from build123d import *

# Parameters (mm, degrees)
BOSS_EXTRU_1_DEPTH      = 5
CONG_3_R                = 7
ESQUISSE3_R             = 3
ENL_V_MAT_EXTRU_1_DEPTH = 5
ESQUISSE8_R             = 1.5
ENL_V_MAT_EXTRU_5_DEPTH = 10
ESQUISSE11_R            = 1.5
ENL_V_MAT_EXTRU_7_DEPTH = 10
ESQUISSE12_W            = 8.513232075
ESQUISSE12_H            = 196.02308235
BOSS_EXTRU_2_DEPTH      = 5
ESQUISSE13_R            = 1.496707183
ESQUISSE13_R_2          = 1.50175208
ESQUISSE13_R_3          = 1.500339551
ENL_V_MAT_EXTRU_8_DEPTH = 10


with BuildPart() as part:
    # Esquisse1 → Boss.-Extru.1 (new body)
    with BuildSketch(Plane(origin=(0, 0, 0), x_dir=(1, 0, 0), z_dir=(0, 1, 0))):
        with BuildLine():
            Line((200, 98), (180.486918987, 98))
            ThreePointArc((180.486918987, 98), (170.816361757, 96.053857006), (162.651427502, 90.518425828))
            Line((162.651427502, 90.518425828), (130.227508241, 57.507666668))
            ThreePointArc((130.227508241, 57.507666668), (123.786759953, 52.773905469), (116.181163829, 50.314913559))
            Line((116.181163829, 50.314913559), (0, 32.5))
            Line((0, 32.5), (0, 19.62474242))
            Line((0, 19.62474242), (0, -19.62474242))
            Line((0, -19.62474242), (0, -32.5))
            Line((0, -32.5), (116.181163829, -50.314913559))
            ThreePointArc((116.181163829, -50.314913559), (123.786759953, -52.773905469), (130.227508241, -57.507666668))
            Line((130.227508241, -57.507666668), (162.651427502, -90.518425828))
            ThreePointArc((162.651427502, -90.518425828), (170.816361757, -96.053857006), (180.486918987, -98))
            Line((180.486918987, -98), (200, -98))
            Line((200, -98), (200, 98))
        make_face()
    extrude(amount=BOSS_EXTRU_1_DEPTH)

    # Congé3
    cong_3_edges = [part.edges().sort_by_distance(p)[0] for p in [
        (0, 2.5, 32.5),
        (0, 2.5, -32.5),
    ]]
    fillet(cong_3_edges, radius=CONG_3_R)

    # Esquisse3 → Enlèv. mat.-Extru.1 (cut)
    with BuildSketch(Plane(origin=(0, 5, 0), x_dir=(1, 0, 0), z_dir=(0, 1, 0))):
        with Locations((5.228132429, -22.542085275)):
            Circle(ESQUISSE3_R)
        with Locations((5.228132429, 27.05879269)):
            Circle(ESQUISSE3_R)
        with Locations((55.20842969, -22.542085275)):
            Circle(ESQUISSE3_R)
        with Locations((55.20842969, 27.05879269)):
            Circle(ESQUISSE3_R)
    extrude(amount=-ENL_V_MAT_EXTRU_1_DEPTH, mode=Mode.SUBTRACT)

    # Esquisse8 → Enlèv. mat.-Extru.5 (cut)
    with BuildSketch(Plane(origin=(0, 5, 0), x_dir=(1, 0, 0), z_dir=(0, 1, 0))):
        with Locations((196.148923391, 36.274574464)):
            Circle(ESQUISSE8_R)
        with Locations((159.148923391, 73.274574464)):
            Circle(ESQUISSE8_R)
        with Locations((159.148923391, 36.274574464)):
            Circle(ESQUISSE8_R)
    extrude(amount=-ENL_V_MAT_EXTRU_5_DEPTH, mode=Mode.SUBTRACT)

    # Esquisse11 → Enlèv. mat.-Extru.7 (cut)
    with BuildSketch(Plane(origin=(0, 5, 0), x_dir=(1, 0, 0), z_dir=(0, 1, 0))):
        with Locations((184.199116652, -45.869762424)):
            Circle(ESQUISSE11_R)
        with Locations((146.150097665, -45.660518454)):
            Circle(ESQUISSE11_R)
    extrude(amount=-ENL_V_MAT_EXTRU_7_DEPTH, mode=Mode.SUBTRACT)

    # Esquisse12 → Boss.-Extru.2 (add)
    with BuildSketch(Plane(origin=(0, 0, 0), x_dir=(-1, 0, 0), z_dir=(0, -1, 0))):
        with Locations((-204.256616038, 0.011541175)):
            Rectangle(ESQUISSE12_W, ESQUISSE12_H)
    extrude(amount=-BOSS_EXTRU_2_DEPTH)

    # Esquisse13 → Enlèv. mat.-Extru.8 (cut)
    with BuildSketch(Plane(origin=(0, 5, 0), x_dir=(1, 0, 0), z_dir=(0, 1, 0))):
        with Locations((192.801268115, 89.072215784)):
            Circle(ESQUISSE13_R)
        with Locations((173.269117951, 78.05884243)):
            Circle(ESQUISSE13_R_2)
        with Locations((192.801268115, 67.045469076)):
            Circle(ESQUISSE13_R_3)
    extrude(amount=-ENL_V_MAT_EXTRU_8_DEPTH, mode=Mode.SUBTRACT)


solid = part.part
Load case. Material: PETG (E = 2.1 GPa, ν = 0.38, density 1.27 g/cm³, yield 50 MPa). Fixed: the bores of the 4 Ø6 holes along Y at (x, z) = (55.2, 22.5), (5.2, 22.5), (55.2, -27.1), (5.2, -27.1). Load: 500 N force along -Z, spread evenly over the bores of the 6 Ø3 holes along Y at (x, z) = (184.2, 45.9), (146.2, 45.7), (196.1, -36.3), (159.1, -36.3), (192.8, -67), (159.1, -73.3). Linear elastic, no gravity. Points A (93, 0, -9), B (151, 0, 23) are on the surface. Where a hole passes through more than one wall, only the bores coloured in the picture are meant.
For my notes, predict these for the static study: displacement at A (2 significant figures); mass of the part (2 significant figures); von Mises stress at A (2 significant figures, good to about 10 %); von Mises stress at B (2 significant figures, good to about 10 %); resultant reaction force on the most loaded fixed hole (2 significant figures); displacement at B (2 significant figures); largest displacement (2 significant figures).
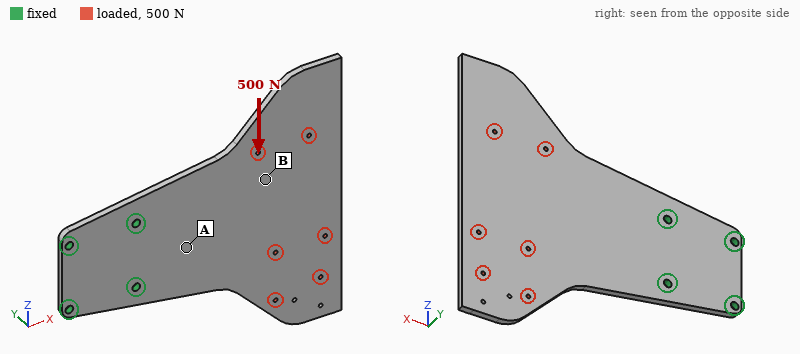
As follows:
0.20 mm
160 g
3.9 MPa
1.8 MPa
970 N
0.65 mm
1.3 mm
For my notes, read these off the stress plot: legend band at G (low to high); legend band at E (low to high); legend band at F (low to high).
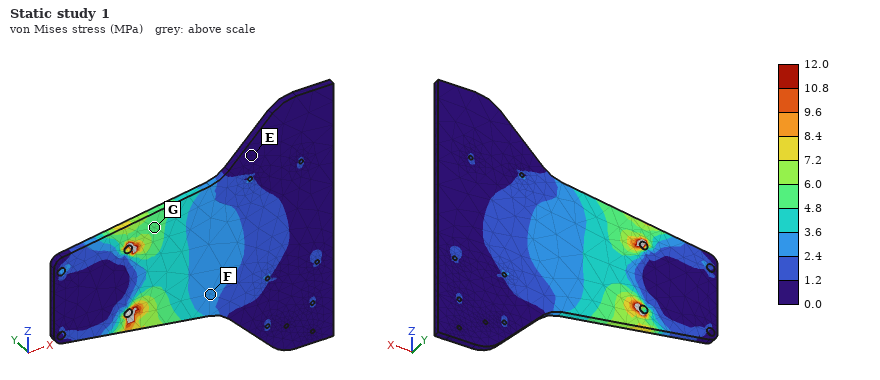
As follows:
4.8 to 6.0 MPa
0.0 to 1.2 MPa
2.4 to 3.6 MPa
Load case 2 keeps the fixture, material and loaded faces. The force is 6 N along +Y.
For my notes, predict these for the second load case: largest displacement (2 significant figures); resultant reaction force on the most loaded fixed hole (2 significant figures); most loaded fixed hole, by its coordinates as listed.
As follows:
2.7 mm
6.2 N
(55.2, -27.1)
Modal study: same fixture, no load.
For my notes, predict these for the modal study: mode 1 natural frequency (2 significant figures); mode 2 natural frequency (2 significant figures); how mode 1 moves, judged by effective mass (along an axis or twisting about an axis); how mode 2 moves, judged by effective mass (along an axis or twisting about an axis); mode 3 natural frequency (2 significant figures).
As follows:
32 Hz
62 Hz
along Y
twisting about X
220 Hz
